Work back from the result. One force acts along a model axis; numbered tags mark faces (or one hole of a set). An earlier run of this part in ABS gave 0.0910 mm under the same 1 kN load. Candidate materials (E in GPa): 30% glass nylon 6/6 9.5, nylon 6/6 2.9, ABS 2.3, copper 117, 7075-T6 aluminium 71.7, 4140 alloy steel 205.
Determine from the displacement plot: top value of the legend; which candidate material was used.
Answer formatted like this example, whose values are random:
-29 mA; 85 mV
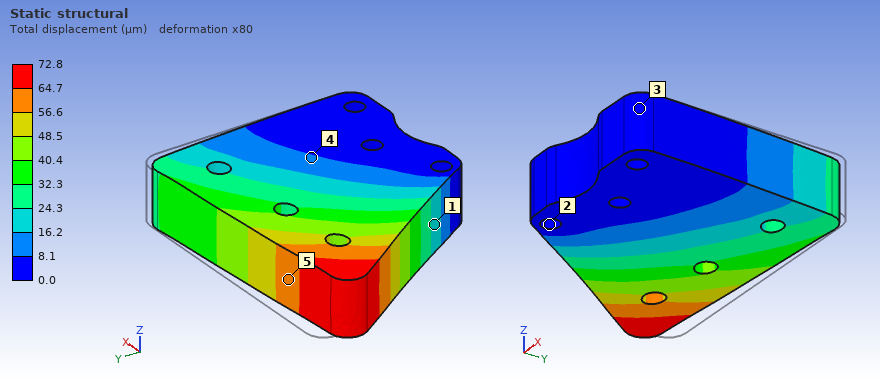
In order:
72.8 µm; nylon 6/6
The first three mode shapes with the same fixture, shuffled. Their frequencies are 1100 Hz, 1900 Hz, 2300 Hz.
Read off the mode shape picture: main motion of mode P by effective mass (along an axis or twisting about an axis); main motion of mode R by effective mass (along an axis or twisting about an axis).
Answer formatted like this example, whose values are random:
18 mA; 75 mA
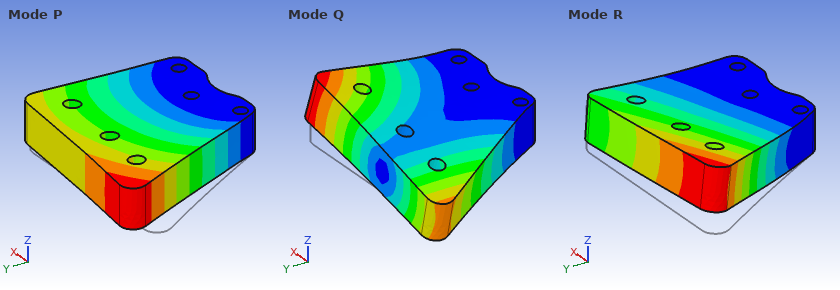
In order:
along X; along Z
